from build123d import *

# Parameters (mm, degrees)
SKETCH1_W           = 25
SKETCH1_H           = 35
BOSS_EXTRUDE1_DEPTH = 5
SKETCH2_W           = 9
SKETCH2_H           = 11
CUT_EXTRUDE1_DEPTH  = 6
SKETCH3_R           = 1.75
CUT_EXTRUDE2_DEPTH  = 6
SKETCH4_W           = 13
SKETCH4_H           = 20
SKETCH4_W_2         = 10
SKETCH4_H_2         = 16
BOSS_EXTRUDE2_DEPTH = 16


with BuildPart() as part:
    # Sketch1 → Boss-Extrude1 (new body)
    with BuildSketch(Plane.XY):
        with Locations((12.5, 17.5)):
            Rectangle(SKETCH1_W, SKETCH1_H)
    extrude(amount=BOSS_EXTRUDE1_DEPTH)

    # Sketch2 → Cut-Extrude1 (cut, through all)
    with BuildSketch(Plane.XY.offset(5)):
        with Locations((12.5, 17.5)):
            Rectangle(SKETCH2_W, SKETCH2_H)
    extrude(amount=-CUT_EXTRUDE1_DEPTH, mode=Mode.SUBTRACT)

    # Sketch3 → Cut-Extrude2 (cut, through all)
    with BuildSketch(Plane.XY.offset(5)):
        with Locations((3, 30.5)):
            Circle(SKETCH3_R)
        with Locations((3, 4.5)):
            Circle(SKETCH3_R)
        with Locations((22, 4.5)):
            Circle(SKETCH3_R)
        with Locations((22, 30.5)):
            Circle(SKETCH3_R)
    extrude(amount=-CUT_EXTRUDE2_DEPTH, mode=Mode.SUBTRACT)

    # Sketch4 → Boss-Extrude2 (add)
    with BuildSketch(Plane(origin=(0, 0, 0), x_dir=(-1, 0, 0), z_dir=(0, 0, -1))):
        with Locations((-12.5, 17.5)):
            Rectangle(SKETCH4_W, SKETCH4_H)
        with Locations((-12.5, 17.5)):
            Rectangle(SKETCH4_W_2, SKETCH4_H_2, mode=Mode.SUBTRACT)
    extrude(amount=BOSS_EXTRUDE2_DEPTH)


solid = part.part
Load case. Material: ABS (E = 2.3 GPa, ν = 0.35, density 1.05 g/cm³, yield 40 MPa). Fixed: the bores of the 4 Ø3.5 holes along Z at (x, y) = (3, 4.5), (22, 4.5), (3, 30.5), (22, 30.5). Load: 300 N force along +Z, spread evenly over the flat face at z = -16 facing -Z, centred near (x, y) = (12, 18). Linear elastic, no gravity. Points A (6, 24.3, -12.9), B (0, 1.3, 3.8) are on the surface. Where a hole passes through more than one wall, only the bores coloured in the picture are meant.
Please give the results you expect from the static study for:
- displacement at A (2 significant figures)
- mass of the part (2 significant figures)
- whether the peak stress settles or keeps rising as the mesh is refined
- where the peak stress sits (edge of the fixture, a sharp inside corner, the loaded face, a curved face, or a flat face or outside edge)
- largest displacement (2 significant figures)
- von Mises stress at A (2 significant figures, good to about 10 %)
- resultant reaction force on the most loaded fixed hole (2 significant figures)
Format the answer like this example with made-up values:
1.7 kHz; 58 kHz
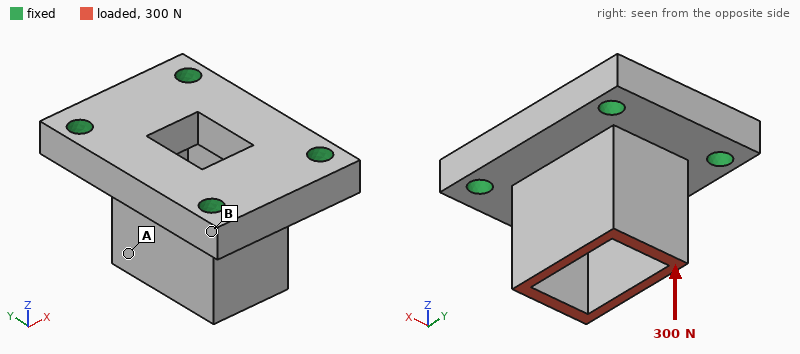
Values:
42 µm; 5.6 g; keeps rising; edge of the fixture; 46 µm; 3.0 MPa; 78 N
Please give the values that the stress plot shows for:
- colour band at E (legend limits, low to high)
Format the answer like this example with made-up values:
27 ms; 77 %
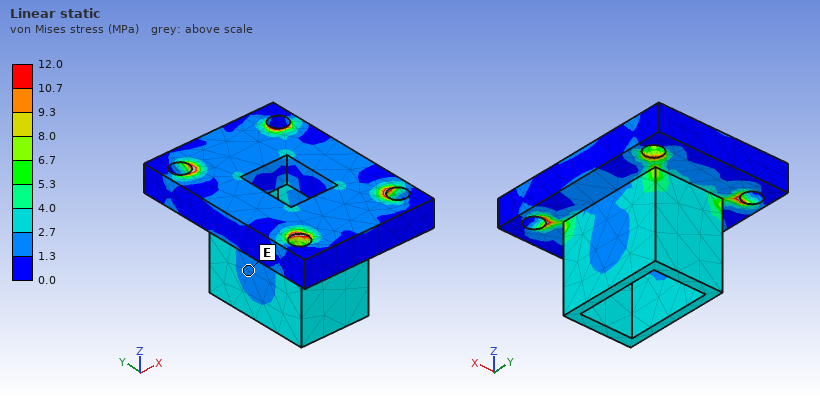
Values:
1.3 to 2.7 MPa
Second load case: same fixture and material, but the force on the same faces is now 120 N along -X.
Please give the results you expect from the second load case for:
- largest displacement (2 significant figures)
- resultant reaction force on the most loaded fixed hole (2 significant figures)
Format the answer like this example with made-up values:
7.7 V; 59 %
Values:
0.36 mm; 75 N
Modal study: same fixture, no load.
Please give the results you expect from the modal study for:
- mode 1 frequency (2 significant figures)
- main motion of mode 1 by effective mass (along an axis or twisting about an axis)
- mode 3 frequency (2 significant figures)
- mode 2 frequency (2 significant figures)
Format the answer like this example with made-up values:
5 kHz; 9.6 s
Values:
5100 Hz; along X; 6800 Hz; 6100 Hz
